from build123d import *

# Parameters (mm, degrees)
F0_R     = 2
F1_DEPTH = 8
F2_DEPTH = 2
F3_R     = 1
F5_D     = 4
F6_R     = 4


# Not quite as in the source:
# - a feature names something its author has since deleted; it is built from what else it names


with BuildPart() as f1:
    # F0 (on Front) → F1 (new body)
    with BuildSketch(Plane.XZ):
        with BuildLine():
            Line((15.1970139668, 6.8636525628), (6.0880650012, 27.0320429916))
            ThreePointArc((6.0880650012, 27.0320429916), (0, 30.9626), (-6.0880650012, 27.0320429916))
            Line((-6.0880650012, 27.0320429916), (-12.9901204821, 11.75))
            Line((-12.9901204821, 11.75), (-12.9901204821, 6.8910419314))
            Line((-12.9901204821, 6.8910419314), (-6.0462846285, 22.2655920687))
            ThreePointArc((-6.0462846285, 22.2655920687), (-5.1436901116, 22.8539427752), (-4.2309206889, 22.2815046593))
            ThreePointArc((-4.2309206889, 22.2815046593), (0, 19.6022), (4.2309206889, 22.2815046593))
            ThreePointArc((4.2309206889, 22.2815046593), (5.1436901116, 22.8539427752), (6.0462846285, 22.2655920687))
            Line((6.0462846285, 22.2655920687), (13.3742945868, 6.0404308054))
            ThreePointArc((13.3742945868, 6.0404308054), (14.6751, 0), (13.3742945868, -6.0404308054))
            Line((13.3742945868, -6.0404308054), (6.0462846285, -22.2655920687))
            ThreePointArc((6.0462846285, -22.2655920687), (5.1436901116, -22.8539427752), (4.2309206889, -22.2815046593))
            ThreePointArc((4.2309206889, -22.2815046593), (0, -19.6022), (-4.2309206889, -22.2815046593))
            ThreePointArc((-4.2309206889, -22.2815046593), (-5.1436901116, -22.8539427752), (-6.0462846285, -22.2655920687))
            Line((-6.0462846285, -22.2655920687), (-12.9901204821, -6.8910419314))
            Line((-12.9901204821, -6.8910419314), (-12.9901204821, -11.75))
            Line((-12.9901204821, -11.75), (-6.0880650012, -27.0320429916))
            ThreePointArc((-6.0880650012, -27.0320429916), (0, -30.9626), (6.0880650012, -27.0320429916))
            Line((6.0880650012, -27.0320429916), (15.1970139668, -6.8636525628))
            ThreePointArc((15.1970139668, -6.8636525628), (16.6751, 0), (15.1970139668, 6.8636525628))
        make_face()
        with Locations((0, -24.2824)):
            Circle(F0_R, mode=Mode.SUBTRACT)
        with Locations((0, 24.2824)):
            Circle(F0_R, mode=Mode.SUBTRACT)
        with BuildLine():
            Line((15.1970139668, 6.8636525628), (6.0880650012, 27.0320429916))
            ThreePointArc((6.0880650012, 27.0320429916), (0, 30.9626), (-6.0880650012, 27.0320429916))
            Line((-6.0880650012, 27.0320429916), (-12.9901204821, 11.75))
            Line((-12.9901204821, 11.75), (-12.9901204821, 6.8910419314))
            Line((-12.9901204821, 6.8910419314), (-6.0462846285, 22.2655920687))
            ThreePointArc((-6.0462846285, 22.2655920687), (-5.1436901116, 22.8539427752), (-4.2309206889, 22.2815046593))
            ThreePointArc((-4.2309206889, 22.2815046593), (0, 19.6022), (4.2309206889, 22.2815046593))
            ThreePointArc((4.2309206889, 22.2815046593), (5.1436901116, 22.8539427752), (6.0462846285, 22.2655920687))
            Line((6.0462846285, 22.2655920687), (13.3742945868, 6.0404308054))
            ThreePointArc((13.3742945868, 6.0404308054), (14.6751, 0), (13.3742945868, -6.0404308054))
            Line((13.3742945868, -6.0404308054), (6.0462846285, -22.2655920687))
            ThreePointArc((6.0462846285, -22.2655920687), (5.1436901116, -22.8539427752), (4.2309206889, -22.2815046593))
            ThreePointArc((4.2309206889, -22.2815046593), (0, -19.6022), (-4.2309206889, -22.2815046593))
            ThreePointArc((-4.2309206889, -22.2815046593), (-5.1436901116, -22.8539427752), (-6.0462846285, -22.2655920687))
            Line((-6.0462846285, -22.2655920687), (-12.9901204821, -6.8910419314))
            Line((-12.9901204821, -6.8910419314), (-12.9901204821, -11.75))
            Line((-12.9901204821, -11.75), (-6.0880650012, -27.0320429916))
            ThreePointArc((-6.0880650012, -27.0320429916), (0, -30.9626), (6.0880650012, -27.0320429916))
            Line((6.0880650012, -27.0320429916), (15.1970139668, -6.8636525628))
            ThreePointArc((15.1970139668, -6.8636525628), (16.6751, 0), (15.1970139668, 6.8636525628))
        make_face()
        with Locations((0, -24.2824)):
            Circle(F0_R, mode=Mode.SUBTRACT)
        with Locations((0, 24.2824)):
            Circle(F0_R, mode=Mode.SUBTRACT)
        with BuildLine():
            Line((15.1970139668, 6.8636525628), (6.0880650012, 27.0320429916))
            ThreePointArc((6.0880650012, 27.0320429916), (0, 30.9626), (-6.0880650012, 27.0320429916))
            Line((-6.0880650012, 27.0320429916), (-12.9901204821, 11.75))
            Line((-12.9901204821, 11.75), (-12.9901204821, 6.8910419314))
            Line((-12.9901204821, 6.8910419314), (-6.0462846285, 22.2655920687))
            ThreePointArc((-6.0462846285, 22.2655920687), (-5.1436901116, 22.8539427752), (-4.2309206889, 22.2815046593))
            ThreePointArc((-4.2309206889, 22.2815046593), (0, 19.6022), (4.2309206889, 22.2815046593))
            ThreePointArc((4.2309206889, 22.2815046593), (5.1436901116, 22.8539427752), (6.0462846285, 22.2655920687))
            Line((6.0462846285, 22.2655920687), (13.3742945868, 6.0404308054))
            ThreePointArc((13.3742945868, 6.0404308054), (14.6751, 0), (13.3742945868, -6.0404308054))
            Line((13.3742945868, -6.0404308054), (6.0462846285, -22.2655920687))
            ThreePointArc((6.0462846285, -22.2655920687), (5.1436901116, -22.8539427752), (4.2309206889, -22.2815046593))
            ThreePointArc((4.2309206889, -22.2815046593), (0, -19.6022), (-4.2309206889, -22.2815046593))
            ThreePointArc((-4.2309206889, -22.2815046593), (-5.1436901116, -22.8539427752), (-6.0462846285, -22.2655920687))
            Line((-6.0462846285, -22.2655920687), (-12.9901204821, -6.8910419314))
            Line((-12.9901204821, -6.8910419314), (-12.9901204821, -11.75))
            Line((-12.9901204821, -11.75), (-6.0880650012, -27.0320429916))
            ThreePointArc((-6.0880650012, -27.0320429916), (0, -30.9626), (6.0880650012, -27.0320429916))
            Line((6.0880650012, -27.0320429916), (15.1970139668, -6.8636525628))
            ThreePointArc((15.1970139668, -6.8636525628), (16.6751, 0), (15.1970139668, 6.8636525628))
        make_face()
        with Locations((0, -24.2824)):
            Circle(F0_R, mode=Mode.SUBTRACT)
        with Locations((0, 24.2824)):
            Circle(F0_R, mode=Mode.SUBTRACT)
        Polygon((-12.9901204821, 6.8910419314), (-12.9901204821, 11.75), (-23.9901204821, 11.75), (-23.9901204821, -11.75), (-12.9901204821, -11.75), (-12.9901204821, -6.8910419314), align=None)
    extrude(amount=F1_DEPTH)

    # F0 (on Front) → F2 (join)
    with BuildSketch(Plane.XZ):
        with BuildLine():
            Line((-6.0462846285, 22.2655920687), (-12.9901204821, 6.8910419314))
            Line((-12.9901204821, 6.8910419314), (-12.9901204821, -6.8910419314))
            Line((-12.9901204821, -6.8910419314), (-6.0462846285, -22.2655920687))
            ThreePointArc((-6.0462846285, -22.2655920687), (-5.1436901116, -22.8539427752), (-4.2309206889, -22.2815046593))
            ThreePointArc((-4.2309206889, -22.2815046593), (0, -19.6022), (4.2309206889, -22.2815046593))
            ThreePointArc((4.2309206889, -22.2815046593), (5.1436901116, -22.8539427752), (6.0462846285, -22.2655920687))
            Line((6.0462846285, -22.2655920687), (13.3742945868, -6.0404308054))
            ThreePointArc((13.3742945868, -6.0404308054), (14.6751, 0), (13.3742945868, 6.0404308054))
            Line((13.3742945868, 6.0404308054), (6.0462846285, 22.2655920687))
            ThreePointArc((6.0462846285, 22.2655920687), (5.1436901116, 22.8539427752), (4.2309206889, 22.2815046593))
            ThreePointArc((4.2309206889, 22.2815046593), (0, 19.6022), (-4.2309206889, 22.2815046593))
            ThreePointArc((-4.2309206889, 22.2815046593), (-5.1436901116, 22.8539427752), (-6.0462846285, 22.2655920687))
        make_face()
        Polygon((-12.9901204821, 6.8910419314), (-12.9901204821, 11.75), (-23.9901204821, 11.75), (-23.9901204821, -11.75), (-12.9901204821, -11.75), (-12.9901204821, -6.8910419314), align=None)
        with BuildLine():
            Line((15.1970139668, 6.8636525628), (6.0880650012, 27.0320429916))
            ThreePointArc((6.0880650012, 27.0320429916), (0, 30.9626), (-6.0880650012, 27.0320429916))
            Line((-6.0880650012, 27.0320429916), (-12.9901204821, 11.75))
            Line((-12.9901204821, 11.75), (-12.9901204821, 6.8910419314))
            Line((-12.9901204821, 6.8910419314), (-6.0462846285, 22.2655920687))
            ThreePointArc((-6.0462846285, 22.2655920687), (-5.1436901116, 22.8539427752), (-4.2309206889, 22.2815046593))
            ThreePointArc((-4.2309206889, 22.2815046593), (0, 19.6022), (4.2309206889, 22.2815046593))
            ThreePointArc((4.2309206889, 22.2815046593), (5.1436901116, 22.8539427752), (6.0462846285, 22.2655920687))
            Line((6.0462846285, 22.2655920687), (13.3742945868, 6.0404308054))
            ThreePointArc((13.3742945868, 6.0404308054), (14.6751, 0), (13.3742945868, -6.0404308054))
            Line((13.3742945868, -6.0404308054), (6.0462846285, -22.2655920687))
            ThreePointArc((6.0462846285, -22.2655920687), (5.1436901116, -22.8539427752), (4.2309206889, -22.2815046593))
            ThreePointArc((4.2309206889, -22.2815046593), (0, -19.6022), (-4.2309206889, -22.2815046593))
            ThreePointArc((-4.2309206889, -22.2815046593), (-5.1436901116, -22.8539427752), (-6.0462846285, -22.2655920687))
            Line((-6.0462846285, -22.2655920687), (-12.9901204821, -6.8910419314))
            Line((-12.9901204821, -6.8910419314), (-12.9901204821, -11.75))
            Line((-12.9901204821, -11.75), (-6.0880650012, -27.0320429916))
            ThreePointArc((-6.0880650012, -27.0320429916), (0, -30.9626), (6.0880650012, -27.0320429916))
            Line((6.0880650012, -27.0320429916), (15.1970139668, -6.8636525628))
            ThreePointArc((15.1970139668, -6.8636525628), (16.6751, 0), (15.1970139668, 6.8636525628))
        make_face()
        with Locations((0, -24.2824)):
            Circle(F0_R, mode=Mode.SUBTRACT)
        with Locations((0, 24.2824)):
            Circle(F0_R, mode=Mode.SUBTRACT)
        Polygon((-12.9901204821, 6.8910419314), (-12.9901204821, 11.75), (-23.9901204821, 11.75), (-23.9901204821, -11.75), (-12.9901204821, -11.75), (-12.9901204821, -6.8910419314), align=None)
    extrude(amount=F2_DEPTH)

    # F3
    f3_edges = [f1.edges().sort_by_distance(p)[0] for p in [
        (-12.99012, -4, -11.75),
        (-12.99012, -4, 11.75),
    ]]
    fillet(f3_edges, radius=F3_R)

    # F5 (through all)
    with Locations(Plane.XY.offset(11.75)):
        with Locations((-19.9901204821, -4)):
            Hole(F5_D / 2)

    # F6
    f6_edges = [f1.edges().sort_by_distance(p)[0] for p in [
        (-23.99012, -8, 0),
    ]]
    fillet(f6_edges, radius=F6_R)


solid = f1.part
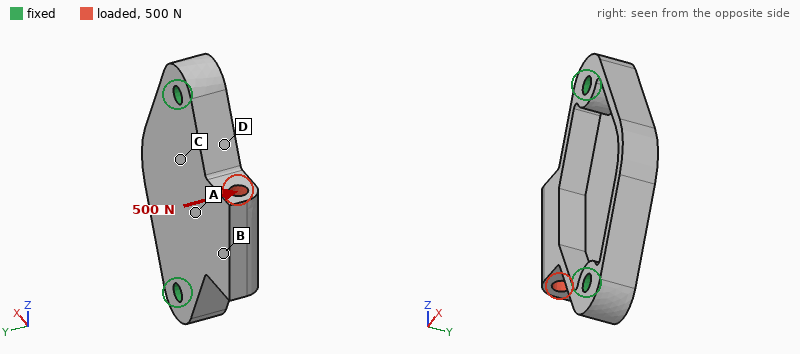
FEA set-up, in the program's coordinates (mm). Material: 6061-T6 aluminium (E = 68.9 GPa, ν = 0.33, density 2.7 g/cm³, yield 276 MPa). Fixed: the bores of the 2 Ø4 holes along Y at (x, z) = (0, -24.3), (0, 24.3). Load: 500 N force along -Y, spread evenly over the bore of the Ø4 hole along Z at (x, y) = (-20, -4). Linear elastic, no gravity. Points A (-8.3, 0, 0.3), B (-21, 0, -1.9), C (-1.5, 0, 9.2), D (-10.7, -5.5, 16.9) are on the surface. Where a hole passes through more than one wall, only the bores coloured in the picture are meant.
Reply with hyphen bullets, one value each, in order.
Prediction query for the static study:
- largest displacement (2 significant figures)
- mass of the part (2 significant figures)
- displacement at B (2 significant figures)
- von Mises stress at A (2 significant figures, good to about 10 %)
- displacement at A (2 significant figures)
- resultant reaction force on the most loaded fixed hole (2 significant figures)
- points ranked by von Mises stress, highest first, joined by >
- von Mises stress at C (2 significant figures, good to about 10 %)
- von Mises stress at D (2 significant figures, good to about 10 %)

- 0.22 mm
- 17 g
- 0.19 mm
- 58 MPa
- 0.045 mm
- 580 N
- D > A > C > B
- 35 MPa
- 140 MPa
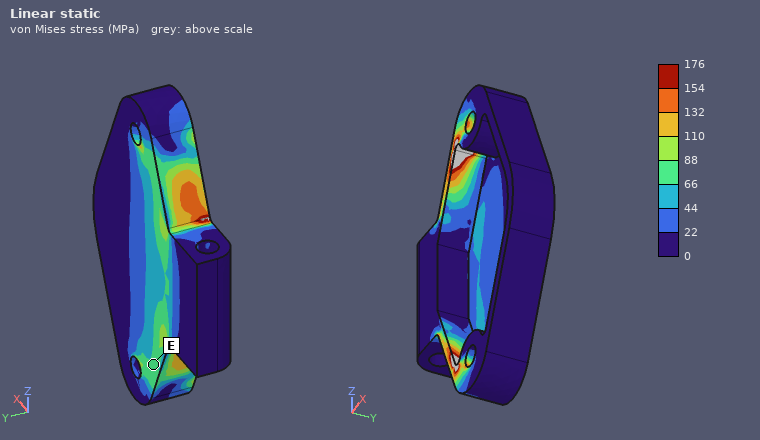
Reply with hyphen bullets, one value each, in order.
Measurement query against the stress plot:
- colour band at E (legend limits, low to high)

- 66 to 88 MPa
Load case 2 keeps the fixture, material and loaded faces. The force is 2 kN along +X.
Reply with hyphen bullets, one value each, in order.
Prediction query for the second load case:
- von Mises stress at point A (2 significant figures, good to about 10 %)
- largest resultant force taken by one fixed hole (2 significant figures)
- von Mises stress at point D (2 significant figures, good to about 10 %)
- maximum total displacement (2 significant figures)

- 43 MPa
- 1.3 kN
- 130 MPa
- 0.17 mm
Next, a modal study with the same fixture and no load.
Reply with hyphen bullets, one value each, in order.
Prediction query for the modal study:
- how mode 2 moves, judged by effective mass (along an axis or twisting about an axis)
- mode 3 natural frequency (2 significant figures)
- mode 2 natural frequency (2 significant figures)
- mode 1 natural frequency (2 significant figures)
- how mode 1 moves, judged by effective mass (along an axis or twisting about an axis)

- along Y
- 12 kHz
- 8900 Hz
- 4200 Hz
- along Y
